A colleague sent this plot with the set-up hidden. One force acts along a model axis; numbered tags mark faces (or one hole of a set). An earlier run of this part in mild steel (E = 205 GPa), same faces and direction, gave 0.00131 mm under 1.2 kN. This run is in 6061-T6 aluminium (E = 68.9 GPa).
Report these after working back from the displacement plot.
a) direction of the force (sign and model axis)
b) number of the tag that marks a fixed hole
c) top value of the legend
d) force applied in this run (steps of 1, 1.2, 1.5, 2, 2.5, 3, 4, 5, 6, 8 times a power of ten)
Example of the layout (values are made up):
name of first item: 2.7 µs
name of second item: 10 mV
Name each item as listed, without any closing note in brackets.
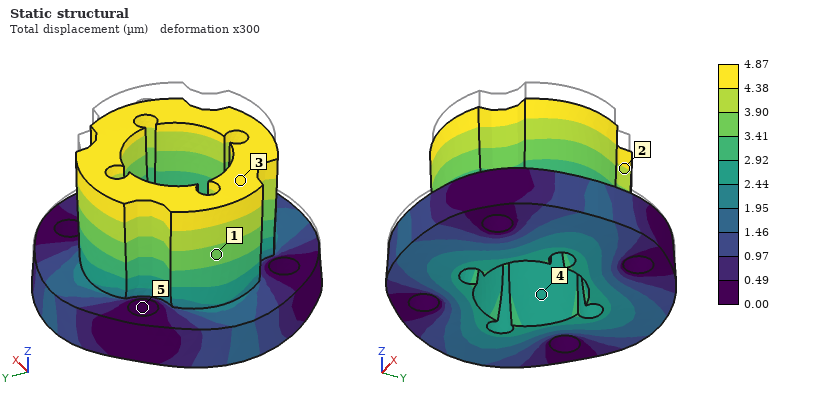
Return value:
direction of the force: -Z
number of the tag that marks a fixed hole: 5
top value of the legend: 4.87 µm
force applied in this run: 1.5 kN
